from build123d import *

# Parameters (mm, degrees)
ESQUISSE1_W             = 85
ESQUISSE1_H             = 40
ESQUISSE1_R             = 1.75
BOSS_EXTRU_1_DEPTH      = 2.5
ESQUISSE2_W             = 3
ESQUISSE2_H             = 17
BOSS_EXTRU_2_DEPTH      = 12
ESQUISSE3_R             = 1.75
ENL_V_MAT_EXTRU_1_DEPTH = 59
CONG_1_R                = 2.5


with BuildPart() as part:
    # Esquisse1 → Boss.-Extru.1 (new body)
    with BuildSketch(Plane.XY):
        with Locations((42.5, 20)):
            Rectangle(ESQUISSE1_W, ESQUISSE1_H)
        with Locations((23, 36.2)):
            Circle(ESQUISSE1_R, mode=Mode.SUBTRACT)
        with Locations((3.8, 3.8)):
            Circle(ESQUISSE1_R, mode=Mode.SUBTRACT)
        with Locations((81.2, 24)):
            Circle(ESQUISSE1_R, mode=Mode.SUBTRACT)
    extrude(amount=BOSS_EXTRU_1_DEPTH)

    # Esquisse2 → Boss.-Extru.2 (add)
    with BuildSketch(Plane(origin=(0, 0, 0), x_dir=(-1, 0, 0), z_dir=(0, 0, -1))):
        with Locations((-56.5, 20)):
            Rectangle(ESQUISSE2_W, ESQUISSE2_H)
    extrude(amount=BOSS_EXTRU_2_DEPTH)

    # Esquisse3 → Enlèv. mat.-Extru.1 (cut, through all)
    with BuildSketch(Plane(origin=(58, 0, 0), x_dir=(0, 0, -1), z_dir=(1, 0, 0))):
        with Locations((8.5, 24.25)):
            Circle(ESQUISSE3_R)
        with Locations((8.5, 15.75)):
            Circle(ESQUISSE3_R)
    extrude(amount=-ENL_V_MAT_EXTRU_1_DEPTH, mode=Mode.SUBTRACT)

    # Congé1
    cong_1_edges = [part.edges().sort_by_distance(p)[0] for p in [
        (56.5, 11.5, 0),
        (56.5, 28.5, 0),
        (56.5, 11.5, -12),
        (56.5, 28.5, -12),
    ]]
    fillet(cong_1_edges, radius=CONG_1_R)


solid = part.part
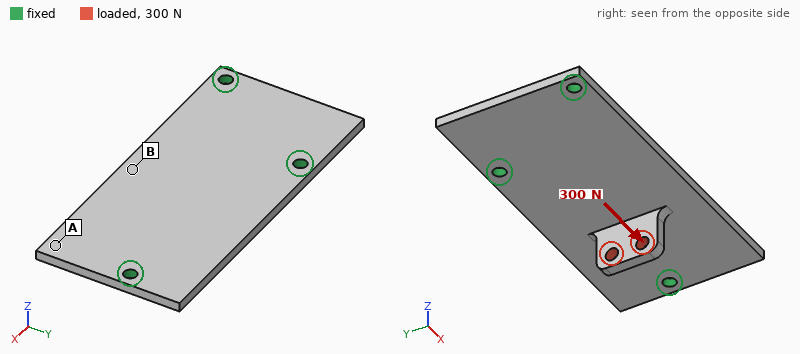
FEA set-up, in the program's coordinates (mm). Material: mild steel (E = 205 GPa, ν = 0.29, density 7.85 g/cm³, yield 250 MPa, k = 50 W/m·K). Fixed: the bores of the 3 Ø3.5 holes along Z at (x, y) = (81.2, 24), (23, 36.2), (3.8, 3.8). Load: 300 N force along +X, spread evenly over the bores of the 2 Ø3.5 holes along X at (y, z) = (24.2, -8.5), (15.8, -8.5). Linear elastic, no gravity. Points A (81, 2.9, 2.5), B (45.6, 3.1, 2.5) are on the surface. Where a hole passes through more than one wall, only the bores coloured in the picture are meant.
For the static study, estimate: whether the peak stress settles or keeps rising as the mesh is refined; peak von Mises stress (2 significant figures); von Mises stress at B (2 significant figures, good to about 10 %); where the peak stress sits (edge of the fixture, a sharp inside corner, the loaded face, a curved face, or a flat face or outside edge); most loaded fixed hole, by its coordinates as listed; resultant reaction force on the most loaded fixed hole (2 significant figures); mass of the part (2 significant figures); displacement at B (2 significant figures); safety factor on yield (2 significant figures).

settles
120 MPa
20 MPa
a curved face
(81.2, 24)
160 N
71 g
17 µm
2.0
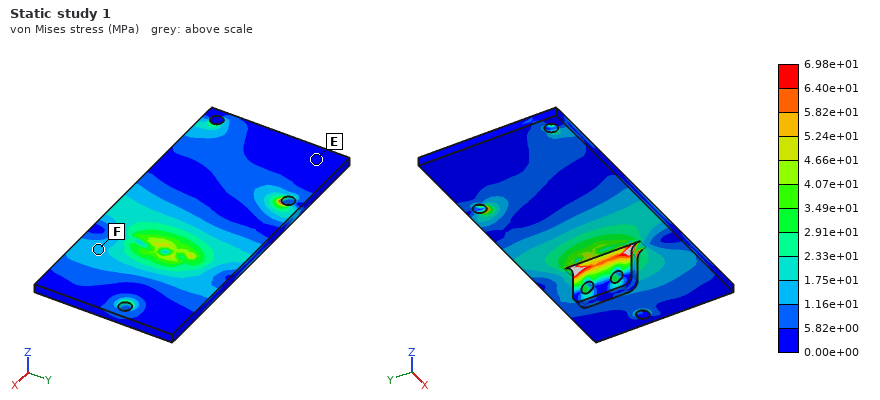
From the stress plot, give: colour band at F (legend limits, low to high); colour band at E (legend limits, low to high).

1.16e+01 to 1.75e+01 MPa
0.00e+00 to 5.82e+00 MPa
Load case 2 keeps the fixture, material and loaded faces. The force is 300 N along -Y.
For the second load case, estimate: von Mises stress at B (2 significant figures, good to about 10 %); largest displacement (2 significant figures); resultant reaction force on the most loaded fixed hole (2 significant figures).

22 MPa
58 µm
150 N
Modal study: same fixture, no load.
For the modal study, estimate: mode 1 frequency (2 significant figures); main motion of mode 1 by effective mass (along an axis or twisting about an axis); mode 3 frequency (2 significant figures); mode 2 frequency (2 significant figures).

2000 Hz
along Z
4800 Hz
3500 Hz
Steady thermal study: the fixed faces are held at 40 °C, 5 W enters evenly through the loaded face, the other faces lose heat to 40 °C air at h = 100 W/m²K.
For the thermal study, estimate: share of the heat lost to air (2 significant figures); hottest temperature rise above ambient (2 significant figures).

69 %
29 K
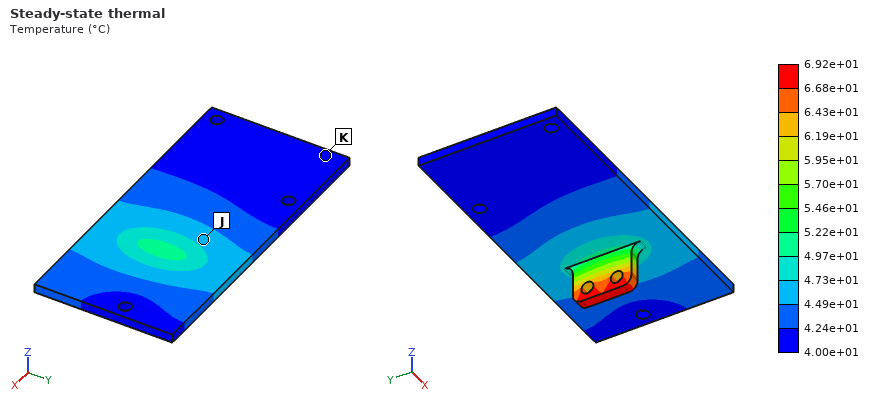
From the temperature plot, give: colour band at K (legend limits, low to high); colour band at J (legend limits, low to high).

4.00e+01 to 4.24e+01 °C
4.49e+01 to 4.73e+01 °C
